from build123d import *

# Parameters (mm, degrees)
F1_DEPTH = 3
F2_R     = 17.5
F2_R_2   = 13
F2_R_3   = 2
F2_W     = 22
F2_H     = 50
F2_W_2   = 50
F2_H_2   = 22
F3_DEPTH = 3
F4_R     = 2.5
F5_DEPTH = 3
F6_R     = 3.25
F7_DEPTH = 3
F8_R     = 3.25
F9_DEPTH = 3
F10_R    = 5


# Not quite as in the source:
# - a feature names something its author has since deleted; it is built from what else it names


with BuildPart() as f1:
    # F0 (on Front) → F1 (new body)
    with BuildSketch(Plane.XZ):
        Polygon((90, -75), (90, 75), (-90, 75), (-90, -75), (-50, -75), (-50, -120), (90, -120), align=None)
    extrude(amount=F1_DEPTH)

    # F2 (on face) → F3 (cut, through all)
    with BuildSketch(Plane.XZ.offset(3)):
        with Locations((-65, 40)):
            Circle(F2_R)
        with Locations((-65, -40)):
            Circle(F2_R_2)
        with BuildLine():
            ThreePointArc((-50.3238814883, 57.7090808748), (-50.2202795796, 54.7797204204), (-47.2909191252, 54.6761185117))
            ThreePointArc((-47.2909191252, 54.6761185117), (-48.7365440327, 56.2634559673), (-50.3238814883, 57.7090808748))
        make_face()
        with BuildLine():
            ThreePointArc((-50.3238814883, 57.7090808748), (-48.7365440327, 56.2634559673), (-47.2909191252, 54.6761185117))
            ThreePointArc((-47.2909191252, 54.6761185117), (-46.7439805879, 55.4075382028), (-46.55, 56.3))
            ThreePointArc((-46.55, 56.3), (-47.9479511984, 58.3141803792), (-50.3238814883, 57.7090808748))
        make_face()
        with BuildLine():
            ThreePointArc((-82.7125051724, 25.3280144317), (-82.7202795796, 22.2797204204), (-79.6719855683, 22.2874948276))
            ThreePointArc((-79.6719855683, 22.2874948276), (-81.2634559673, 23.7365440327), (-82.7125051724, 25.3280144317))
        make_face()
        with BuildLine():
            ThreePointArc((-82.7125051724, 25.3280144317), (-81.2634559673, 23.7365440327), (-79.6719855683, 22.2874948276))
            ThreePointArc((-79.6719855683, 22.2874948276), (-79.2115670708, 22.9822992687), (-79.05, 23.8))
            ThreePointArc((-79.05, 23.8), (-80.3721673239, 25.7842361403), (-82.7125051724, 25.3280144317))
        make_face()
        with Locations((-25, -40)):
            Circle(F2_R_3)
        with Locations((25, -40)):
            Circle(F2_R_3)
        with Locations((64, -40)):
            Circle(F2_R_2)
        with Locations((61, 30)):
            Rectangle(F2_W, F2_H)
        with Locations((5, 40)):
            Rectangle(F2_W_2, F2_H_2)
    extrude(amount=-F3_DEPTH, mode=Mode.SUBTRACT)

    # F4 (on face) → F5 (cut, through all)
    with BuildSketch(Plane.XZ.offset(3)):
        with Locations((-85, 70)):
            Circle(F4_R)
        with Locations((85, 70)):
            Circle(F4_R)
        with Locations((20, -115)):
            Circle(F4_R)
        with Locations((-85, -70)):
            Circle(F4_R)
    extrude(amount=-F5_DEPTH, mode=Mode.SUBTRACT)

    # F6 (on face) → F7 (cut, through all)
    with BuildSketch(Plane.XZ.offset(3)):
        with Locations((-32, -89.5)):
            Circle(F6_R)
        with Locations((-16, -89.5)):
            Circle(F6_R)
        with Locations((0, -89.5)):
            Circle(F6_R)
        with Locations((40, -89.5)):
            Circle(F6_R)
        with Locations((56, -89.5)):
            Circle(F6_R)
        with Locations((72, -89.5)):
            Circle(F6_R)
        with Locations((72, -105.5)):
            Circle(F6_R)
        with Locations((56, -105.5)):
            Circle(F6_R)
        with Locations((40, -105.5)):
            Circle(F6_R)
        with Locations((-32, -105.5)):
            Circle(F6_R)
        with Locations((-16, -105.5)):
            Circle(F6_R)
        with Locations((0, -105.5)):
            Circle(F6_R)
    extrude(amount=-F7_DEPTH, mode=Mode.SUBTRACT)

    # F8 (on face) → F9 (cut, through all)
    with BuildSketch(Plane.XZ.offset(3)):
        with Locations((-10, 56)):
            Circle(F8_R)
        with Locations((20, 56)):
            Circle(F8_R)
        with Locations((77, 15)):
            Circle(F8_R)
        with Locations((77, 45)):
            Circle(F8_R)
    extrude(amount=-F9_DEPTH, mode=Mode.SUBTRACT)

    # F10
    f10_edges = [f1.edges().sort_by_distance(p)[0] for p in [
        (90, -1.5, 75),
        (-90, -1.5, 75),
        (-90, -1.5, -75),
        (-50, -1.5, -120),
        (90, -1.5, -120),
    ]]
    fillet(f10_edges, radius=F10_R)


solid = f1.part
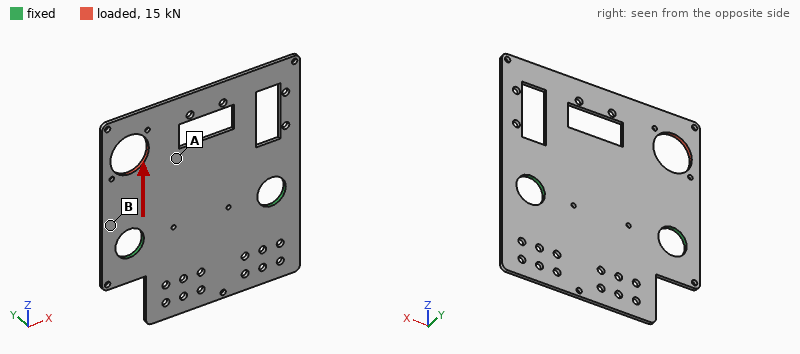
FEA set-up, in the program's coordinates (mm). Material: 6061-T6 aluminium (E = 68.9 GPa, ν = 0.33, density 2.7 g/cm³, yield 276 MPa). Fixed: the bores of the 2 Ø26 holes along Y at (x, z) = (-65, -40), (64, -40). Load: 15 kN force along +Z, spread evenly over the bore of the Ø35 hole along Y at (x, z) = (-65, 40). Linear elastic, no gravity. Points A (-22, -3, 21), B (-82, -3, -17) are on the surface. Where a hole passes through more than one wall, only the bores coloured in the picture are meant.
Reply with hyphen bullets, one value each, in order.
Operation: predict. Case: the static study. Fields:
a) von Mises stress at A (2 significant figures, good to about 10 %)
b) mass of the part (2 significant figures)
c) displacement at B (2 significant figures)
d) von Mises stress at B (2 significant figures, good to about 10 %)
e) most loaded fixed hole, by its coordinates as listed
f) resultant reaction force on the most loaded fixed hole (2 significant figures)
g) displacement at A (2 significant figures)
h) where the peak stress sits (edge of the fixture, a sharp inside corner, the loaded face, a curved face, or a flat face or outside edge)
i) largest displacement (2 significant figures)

- 30 MPa
- 230 g
- 0.032 mm
- 97 MPa
- (-65, -40)
- 15 kN
- 0.036 mm
- a curved face
- 0.21 mm
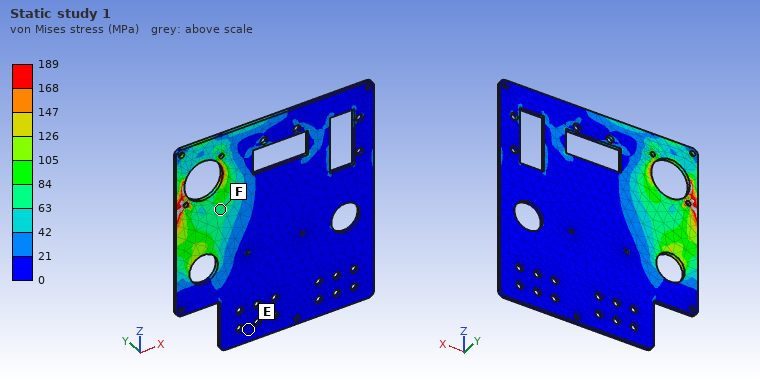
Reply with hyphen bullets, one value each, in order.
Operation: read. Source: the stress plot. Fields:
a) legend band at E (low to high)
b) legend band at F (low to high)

- 0 to 21 MPa
- 63 to 84 MPa
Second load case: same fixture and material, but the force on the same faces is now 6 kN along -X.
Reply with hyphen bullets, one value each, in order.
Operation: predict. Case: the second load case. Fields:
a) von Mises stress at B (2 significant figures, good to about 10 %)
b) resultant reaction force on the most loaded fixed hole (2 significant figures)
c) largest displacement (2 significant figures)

- 33 MPa
- 4.5 kN
- 0.16 mm
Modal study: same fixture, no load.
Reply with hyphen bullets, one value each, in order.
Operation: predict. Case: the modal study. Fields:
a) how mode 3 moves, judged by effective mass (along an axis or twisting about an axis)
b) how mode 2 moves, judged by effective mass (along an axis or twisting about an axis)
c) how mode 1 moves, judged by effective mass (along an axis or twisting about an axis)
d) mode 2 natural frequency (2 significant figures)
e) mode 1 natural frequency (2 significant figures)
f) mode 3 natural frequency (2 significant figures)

- along Y
- twisting about Z
- along Y
- 390 Hz
- 220 Hz
- 450 Hz
